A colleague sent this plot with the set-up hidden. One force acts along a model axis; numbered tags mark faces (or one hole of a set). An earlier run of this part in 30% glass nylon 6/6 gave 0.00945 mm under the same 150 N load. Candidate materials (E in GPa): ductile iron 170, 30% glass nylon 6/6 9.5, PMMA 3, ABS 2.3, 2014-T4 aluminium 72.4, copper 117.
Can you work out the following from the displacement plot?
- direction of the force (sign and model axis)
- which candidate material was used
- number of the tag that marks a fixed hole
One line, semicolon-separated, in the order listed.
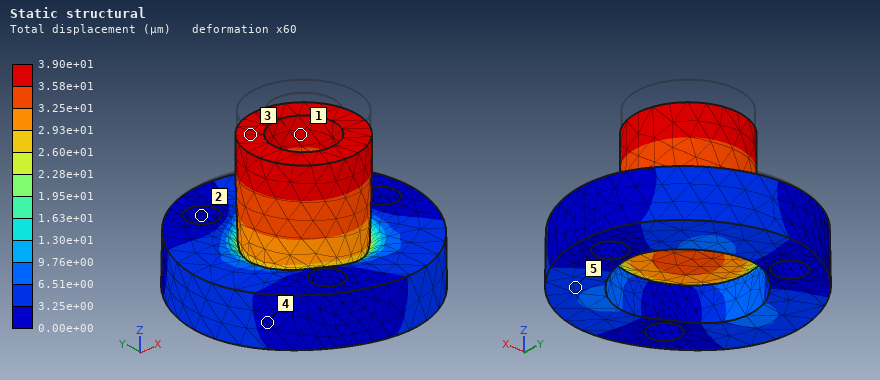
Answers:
-Z; ABS; 2
